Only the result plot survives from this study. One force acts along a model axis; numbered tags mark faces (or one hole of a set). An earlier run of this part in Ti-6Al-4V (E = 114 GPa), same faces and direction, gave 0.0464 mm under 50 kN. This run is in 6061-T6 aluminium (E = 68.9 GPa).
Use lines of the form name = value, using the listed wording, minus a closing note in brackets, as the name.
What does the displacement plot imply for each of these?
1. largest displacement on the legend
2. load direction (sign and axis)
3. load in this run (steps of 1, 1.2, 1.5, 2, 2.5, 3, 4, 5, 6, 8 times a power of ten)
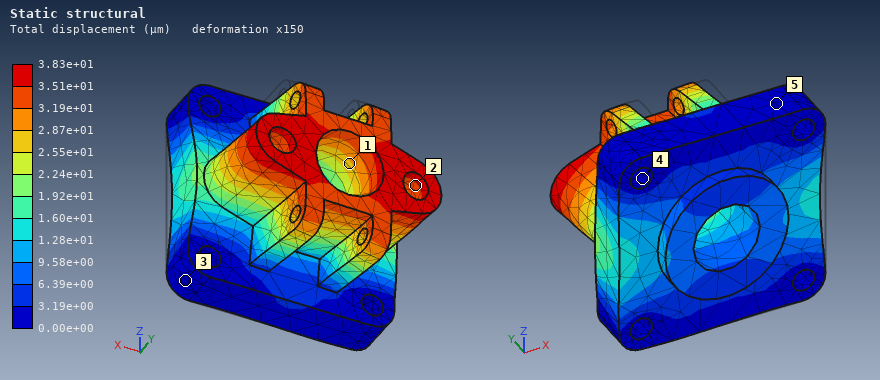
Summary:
largest displacement on the legend = 3.83e+01 µm
load direction = -X
load in this run = 25 kN
